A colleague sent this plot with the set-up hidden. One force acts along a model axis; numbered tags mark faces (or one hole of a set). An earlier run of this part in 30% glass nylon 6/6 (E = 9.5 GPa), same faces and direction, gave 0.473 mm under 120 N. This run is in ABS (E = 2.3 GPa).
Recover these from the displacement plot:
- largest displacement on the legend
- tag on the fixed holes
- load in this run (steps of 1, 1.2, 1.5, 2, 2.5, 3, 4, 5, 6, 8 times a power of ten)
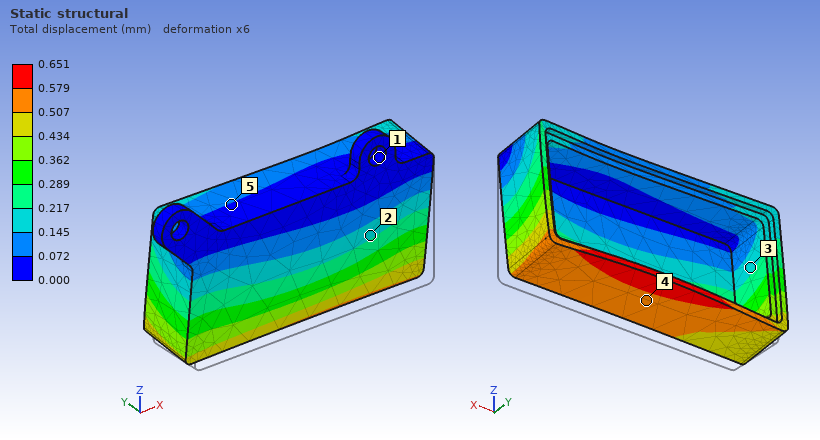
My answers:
0.651 mm
1
40 N
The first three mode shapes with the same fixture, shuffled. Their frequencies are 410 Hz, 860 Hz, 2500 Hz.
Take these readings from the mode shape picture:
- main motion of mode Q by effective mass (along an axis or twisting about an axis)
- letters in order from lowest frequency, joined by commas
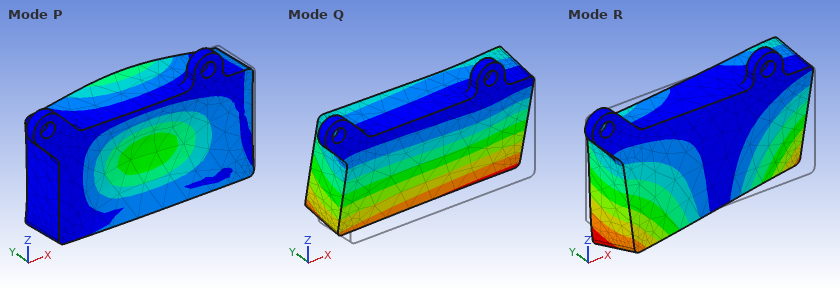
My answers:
along Y
Q, R, P
